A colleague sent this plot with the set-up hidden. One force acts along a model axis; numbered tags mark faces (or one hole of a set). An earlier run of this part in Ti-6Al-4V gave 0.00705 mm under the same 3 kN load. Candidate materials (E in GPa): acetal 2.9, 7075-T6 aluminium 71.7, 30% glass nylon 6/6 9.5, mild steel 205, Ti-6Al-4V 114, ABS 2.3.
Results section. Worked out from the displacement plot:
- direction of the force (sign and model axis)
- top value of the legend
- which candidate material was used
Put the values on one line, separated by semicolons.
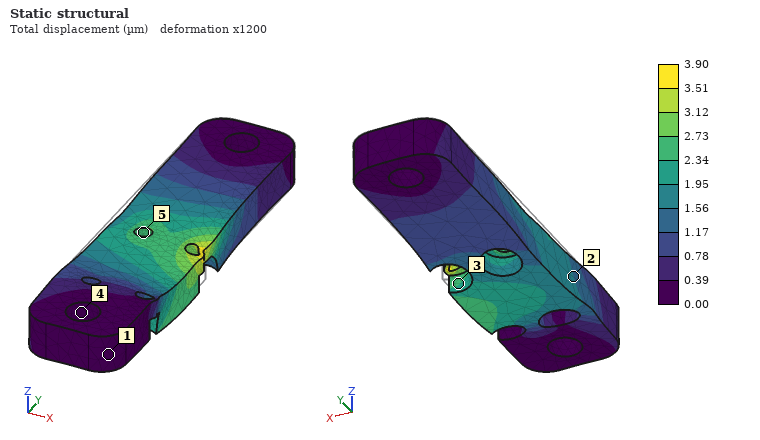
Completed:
-Y; 3.90 µm; mild steel
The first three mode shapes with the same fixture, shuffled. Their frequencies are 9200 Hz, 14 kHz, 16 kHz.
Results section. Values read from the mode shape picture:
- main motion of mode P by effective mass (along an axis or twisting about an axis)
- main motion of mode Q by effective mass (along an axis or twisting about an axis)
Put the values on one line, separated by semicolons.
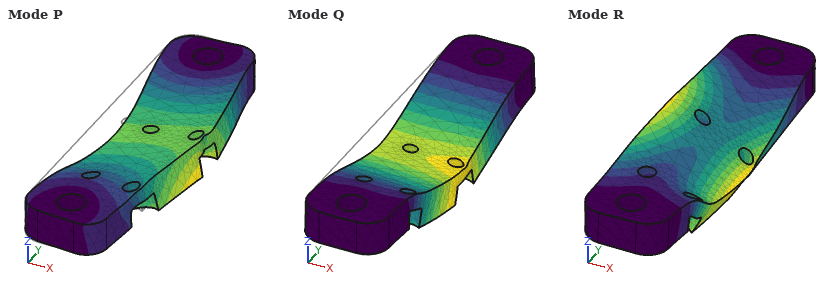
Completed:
along X; along Z
